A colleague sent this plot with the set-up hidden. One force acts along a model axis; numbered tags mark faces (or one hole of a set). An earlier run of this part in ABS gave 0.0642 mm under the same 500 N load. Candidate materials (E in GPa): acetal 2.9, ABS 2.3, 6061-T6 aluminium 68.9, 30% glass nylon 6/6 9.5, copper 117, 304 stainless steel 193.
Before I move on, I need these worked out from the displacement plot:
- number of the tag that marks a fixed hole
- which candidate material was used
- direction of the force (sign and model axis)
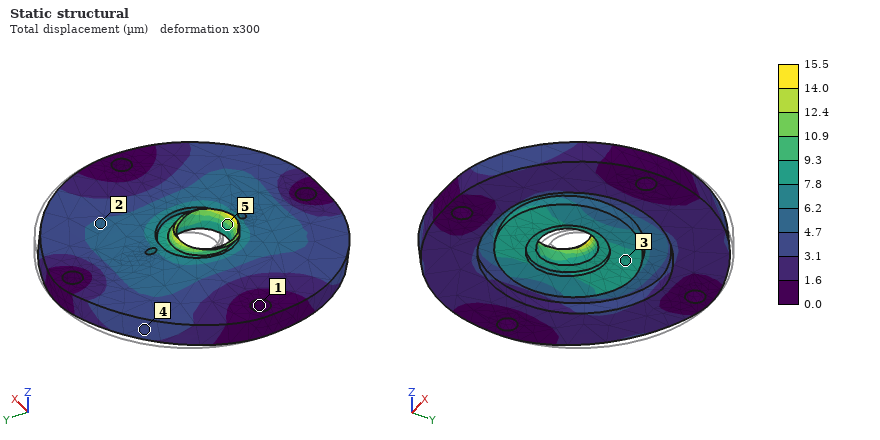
1
30% glass nylon 6/6
-Y
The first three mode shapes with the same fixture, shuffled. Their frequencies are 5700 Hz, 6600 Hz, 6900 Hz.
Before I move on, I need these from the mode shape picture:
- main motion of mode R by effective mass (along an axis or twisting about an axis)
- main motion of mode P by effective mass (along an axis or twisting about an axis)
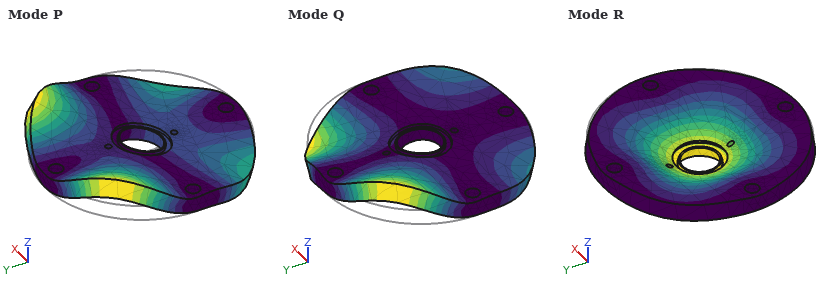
along Z
twisting about X
